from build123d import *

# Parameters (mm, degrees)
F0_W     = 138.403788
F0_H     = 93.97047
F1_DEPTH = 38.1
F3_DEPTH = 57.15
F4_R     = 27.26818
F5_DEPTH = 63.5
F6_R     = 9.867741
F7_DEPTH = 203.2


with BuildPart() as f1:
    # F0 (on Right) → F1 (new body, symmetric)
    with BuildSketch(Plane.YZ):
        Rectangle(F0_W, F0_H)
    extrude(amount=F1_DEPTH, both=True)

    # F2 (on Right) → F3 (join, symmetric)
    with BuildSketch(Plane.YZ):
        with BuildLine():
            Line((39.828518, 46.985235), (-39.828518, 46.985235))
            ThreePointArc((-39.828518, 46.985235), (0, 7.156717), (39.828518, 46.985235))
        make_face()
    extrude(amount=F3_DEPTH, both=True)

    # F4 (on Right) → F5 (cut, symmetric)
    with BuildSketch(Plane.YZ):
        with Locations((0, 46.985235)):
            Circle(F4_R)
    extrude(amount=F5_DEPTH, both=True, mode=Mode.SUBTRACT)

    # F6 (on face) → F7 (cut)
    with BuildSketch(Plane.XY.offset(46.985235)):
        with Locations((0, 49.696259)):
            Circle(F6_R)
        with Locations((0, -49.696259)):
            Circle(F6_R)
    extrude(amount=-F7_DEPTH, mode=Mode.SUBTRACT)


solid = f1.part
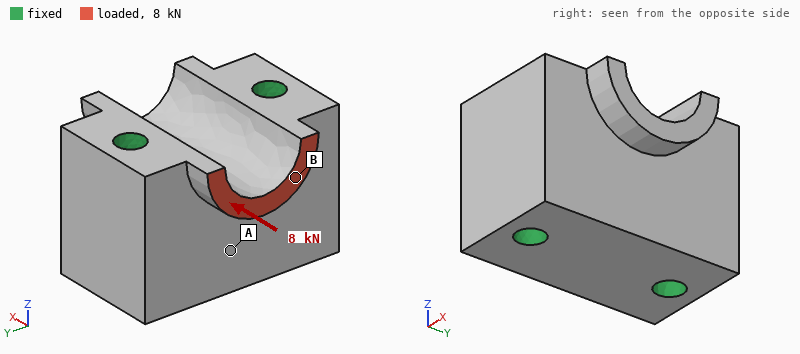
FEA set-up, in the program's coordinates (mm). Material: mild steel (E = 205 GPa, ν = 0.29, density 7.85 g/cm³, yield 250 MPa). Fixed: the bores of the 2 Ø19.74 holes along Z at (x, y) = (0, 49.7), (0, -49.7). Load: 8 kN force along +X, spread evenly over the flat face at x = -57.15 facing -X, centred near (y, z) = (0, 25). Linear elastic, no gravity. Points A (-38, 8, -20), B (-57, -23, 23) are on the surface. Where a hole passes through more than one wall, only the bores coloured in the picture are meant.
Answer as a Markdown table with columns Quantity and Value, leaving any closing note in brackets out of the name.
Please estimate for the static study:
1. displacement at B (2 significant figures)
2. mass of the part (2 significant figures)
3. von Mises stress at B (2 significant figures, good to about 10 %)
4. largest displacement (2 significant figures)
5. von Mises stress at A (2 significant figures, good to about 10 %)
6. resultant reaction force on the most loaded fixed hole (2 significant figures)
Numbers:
| Quantity | Value |
|---|---|
| displacement at B | 1.4 µm |
| mass of the part | 7.0 kg |
| von Mises stress at B | 5.8 MPa |
| largest displacement | 2.0 µm |
| von Mises stress at A | 0.77 MPa |
| resultant reaction force on the most loaded fixed hole | 4.1 kN |
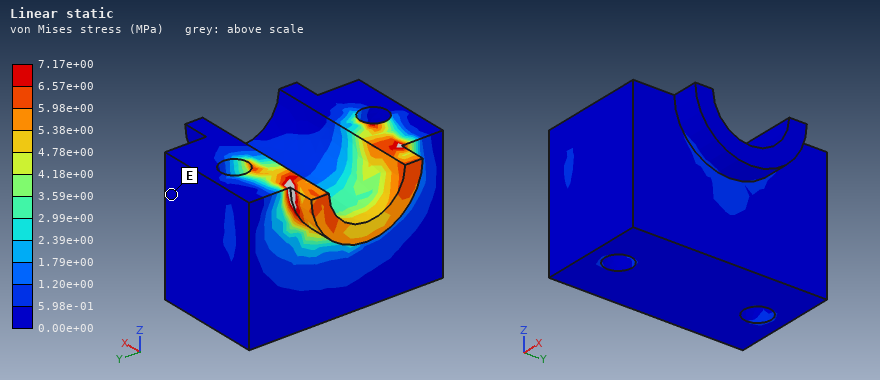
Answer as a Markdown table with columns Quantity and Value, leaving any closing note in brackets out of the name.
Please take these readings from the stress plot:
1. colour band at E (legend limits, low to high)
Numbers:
| Quantity | Value |
|---|---|
| colour band at E | 0.00e+00 to 5.98e-01 MPa |
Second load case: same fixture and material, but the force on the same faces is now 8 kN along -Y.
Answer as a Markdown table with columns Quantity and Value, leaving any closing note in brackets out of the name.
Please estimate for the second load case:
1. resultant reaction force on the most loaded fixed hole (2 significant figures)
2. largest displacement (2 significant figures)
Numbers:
| Quantity | Value |
|---|---|
| resultant reaction force on the most loaded fixed hole | 5.7 kN |
| largest displacement | 11 µm |
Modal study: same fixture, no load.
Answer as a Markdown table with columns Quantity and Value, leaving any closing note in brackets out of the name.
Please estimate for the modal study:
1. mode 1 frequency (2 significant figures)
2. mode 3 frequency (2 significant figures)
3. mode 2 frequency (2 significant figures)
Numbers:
| Quantity | Value |
|---|---|
| mode 1 frequency | 13 kHz |
| mode 3 frequency | 14 kHz |
| mode 2 frequency | 13 kHz |
